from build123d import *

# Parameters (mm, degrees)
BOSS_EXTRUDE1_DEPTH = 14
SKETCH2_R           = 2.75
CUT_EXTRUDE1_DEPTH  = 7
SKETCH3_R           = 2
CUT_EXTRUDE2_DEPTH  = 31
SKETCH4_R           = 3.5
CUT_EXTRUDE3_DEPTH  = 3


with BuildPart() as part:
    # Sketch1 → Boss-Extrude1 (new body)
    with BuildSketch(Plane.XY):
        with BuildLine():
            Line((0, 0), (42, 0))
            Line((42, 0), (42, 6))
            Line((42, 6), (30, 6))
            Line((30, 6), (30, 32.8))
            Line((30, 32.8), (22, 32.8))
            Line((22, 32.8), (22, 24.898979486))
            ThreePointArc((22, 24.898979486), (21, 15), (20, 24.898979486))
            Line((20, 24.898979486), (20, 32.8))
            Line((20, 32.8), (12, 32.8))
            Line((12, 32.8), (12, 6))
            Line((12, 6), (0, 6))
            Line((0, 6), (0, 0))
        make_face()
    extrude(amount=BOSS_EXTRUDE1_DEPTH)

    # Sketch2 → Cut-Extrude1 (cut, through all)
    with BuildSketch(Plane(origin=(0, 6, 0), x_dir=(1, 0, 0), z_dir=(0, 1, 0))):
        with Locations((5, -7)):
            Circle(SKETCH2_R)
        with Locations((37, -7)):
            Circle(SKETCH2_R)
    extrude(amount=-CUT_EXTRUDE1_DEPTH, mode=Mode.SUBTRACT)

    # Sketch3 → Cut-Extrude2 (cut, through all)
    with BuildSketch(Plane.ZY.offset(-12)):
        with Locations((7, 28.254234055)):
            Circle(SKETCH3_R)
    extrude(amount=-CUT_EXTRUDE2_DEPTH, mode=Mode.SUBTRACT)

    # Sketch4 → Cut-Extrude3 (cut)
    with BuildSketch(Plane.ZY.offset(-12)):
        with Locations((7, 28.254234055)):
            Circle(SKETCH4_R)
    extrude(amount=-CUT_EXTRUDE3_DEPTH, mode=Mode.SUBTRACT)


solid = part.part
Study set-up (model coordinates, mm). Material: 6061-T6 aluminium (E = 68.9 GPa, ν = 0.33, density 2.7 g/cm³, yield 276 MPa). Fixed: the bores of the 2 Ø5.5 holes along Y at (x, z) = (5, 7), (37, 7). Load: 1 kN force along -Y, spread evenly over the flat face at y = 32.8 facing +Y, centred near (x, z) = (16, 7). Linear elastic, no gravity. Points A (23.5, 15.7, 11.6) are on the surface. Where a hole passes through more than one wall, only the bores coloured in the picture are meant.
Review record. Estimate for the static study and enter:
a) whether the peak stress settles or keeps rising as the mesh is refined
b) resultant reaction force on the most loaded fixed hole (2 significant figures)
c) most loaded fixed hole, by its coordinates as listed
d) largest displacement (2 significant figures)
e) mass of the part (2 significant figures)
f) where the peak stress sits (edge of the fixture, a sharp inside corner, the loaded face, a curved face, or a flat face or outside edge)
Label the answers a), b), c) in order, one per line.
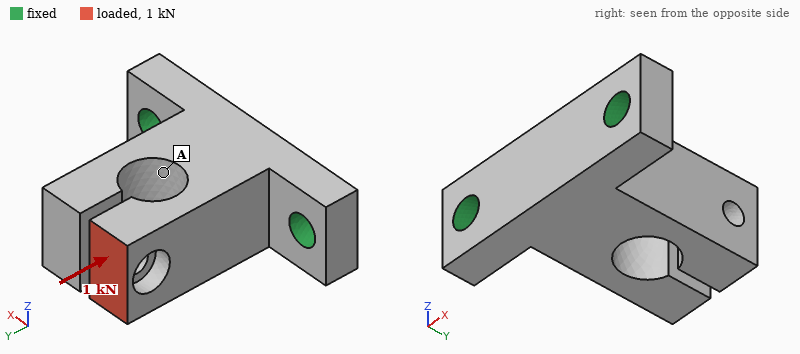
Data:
a) keeps rising
b) 730 N
c) (5, 7)
d) 36 µm
e) 23 g
f) edge of the fixture
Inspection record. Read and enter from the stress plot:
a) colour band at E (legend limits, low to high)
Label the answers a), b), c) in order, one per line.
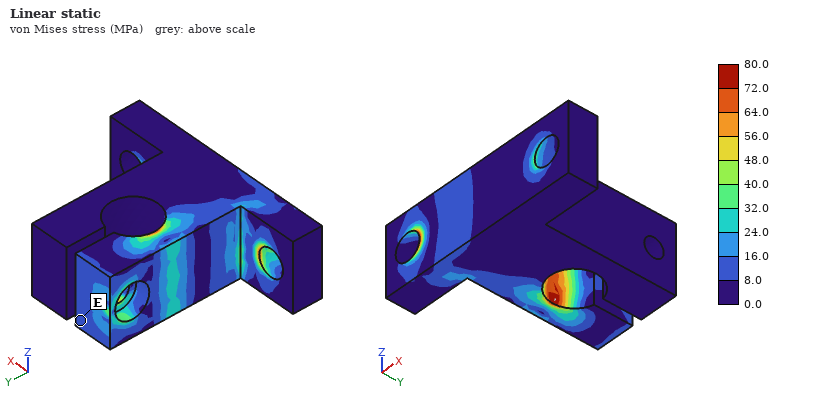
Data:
a) 8.0 to 16.0 MPa
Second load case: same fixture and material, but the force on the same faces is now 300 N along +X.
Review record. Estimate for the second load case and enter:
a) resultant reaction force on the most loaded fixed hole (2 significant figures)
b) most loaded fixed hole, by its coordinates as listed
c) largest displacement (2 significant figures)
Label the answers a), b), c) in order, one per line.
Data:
a) 440 N
b) (37, 7)
c) 0.11 mm
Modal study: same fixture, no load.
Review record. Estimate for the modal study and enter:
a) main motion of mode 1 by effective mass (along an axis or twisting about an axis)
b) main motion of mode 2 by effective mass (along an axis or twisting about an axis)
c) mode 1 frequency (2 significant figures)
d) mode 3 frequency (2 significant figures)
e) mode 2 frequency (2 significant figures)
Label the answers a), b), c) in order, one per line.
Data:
a) along Z
b) along X
c) 5300 Hz
d) 7900 Hz
e) 7100 Hz
